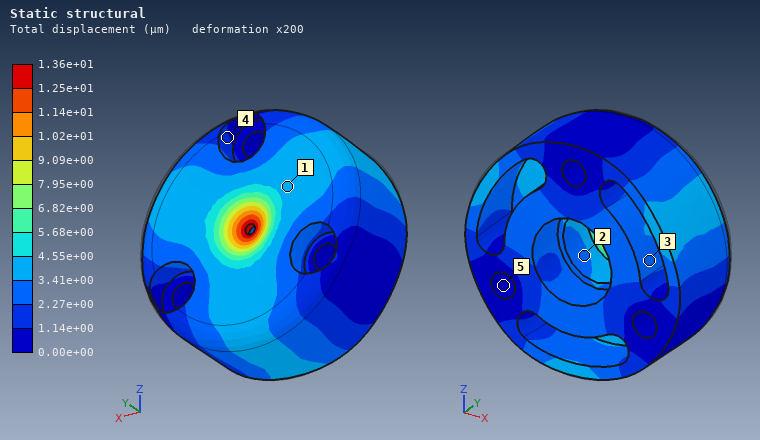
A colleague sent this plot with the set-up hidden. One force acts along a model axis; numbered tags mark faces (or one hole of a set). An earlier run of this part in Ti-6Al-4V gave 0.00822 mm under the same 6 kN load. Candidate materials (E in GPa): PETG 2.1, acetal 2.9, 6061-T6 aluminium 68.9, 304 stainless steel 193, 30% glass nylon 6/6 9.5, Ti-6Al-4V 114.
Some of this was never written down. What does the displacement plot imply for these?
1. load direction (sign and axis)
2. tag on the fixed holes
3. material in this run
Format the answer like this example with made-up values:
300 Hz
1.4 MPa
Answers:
-Y
5
6061-T6 aluminium
